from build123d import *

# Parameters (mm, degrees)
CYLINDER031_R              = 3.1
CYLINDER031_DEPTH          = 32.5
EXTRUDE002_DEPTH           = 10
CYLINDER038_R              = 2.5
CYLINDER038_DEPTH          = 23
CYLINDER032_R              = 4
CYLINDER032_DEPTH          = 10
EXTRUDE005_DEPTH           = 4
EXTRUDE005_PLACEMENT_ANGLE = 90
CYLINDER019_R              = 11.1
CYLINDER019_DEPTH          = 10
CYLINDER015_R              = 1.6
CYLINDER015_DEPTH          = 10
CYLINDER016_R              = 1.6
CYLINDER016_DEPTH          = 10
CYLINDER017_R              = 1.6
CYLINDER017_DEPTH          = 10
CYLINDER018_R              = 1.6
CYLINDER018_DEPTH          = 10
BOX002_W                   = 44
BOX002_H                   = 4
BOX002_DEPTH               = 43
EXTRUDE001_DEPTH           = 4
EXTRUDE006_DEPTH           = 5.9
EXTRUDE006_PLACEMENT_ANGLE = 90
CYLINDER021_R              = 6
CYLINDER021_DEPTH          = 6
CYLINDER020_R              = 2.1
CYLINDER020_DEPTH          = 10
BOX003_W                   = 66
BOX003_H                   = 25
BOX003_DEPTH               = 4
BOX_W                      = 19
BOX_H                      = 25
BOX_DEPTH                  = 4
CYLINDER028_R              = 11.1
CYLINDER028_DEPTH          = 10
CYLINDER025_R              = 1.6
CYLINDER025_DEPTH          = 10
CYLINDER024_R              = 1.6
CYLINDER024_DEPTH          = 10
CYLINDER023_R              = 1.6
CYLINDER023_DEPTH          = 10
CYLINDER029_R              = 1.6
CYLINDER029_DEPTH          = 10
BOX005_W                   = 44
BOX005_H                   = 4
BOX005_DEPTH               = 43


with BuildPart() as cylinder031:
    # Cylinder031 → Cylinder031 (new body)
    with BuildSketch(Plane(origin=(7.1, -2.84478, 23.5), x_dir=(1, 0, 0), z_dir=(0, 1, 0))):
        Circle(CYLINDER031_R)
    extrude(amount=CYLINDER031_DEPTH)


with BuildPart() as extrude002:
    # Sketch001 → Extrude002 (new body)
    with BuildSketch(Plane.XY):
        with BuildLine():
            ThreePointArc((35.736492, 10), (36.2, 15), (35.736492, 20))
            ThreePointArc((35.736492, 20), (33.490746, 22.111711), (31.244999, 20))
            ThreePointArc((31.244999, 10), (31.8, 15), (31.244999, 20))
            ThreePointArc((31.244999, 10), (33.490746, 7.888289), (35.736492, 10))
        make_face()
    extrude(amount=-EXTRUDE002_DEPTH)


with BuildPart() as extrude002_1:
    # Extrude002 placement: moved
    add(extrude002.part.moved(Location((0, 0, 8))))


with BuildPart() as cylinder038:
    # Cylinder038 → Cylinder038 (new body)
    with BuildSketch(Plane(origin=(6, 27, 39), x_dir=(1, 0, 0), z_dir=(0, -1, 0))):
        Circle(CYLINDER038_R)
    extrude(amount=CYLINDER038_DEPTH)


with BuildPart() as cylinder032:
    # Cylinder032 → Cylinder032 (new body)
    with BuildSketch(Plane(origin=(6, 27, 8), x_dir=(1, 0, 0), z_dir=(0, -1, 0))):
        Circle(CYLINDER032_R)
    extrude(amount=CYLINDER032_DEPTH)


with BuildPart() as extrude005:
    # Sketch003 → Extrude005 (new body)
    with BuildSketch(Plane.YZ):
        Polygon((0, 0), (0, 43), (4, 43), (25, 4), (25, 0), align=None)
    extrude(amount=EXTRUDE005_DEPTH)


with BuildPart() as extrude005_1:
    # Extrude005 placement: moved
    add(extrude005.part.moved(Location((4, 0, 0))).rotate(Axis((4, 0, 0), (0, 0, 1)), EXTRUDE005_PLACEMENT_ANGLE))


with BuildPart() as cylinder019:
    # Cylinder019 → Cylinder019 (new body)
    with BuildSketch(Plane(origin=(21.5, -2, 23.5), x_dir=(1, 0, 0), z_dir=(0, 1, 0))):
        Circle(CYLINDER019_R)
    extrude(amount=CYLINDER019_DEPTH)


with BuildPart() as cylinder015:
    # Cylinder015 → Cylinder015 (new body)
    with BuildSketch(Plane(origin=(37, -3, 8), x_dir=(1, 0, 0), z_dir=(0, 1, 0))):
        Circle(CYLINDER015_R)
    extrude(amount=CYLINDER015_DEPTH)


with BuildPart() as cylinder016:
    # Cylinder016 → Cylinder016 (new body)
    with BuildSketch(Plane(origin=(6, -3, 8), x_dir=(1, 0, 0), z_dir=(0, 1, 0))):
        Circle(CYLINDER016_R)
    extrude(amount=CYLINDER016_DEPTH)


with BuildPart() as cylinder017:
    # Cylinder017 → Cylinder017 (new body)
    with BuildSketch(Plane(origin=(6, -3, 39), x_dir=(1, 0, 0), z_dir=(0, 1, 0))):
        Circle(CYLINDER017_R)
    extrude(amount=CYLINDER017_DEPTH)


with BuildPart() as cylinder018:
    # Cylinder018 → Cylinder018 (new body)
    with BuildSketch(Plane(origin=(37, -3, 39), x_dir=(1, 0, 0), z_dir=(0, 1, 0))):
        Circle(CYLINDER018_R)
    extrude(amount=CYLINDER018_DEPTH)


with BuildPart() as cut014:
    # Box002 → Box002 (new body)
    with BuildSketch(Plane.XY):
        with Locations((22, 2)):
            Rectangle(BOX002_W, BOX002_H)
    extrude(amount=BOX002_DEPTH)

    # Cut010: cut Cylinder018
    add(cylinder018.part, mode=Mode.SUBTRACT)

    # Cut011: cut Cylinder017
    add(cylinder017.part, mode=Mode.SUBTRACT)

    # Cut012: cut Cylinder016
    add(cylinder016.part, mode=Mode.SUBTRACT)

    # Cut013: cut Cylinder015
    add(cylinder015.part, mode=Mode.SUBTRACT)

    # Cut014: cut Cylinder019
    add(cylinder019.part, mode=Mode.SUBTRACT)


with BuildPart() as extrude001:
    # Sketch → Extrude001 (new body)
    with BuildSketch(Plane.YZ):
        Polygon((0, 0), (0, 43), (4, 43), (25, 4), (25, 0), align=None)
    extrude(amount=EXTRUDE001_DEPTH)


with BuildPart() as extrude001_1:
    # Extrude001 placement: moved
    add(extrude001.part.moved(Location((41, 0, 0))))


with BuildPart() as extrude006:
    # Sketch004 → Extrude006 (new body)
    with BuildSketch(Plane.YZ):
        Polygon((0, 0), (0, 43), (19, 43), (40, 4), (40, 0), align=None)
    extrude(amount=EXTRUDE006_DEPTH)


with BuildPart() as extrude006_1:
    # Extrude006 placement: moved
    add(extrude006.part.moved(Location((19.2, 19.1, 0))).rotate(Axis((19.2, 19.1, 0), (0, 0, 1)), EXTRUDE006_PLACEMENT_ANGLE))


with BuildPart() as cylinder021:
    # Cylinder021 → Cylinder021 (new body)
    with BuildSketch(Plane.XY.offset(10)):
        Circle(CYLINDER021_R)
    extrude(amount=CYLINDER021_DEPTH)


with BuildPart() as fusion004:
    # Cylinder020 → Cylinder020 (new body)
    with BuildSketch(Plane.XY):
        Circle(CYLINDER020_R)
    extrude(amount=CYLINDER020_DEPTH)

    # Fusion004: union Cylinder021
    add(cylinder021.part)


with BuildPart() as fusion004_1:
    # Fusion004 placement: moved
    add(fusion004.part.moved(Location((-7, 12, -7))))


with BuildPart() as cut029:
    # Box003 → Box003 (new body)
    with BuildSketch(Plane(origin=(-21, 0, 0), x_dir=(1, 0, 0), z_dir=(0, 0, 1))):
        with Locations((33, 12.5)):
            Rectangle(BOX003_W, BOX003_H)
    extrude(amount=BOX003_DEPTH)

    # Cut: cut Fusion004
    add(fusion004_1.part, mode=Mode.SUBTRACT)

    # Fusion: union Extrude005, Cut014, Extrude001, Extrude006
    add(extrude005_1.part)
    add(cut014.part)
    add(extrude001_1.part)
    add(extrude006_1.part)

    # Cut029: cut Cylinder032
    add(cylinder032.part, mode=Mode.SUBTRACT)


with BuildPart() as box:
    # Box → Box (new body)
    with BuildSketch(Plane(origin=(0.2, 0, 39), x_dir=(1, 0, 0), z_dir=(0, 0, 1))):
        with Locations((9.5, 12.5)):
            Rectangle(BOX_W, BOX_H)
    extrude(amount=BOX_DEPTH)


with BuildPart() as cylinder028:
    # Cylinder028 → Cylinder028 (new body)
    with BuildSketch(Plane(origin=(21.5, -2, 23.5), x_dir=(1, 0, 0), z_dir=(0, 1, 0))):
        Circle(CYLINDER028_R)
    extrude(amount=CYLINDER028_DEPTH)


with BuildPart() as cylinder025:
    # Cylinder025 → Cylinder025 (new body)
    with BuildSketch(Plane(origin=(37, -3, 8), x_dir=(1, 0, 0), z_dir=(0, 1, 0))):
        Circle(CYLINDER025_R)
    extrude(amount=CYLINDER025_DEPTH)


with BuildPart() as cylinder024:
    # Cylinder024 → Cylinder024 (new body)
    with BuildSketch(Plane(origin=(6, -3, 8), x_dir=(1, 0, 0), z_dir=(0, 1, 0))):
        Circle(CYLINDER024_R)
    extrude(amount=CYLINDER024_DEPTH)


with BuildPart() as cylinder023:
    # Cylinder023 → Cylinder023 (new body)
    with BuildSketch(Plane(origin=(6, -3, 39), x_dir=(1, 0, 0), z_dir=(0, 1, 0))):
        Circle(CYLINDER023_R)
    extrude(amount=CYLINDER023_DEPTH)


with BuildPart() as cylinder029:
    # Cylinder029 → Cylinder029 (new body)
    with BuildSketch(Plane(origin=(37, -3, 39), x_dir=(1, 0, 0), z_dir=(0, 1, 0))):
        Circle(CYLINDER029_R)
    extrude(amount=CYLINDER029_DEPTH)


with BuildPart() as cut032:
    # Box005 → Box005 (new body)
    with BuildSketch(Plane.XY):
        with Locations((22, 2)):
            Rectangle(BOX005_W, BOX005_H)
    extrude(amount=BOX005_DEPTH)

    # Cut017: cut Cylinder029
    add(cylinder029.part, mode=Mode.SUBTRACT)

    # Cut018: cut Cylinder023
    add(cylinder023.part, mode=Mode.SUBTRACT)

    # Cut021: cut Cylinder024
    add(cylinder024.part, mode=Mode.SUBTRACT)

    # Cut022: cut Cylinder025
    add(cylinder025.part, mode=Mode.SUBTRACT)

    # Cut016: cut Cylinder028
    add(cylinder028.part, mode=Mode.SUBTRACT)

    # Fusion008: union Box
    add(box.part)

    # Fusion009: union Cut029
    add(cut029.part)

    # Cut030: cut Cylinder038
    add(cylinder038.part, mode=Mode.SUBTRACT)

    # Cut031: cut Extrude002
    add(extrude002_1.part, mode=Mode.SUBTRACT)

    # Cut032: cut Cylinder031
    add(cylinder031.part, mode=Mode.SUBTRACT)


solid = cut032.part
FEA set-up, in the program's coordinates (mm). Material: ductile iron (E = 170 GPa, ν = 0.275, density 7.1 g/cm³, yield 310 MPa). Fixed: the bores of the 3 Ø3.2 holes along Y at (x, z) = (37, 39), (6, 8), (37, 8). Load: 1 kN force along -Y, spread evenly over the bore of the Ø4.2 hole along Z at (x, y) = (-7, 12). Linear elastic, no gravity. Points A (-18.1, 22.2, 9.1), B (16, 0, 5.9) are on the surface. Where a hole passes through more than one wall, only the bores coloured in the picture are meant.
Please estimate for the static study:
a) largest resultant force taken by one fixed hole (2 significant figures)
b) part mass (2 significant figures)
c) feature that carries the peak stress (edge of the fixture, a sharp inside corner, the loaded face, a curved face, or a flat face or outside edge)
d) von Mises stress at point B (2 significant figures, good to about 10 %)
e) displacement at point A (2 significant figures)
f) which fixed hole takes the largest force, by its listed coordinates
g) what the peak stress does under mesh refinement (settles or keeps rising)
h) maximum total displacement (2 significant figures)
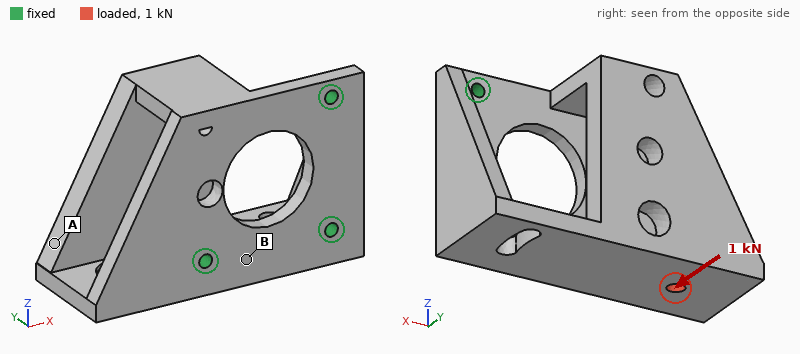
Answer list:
1.4 kN
160 g
edge of the fixture
13 MPa
19 µm
(6, 8)
keeps rising
22 µm
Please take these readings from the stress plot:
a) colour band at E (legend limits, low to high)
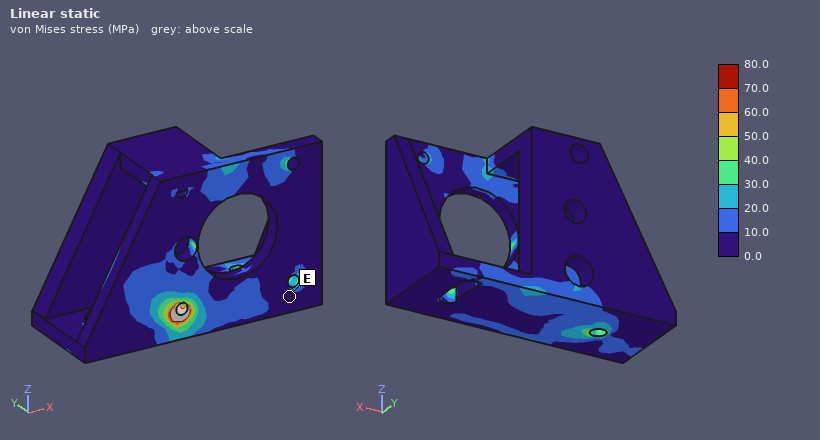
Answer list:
0.0 to 10.0 MPa
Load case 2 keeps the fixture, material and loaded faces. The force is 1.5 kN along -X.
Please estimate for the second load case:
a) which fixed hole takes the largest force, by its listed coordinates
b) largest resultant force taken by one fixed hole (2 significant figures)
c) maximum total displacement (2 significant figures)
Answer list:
(6, 8)
1.1 kN
11 µm
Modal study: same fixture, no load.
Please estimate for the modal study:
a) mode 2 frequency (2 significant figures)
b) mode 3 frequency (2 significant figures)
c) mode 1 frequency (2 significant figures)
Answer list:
3900 Hz
5600 Hz
2600 Hz
